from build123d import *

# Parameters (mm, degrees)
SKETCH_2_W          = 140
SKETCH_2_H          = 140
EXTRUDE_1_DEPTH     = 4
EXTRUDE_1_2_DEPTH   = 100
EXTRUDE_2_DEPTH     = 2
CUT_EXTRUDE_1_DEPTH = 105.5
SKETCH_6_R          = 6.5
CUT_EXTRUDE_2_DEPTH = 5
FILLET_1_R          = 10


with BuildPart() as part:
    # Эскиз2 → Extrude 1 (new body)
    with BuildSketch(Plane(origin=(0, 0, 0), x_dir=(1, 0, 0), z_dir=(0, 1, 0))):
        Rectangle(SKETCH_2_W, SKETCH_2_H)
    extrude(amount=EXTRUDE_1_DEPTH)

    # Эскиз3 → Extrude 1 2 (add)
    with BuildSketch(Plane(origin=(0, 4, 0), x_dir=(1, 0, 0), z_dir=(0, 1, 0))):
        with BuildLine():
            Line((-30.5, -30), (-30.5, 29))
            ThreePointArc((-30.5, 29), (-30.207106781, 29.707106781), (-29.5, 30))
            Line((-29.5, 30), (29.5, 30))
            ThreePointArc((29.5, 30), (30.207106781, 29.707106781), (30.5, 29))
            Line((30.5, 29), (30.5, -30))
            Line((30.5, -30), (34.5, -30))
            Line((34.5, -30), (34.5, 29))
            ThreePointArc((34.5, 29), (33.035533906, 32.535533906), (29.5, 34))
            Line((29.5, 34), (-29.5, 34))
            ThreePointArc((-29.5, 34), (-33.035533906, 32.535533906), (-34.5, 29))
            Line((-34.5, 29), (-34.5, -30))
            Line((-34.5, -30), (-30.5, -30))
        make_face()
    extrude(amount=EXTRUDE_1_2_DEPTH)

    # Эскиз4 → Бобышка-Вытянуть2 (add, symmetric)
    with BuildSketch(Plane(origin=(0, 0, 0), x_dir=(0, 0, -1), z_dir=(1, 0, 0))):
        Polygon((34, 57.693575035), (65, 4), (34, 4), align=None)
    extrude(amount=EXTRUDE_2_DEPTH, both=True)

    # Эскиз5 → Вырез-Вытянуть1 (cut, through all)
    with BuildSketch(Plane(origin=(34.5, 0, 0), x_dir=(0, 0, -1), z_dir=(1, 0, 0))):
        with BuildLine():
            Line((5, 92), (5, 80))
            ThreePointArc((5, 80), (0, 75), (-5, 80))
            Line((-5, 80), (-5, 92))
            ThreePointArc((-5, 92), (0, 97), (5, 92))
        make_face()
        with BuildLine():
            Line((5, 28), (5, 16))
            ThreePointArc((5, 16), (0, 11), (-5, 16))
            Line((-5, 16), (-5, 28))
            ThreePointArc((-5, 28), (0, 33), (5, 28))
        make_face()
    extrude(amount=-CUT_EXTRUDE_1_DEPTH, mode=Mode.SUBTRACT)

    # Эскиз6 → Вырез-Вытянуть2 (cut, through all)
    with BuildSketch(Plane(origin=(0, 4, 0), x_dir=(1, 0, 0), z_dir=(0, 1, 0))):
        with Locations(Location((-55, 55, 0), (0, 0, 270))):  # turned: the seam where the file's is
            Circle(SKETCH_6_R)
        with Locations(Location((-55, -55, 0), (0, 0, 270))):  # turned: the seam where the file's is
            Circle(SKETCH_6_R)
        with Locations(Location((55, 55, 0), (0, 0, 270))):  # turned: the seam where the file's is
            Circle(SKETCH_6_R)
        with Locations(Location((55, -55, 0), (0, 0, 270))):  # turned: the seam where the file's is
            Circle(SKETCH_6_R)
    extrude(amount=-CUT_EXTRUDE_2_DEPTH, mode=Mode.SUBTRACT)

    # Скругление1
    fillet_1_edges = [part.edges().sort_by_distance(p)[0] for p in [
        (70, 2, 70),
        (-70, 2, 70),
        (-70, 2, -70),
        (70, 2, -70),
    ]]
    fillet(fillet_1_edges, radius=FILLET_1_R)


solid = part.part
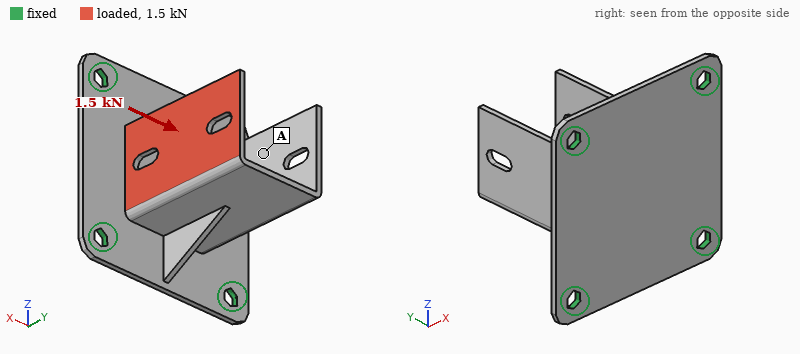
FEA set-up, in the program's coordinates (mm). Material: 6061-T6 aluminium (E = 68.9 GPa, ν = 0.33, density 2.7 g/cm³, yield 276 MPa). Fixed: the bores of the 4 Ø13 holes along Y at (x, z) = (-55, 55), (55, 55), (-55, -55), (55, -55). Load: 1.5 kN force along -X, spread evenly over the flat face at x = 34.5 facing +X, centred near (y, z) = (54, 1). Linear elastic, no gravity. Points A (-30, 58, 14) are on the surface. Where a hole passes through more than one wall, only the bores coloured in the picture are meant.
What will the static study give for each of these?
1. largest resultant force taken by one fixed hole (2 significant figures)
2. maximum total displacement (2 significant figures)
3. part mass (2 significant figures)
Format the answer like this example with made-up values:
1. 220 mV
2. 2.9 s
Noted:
1. 930 N
2. 2.0 mm
3. 410 g
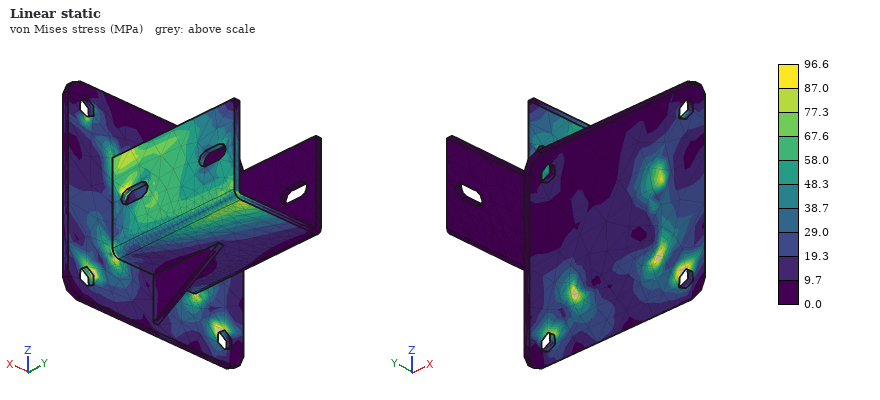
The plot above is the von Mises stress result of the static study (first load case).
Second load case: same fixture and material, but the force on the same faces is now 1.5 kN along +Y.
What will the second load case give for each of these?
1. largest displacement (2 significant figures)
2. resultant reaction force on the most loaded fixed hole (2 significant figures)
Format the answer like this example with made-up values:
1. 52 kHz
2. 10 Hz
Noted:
1. 0.23 mm
2. 690 N
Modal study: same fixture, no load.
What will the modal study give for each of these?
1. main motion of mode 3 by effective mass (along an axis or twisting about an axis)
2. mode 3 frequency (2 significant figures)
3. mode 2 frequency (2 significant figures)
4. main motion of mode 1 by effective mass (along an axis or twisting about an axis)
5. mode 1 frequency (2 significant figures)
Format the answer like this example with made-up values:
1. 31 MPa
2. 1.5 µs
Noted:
1. along Z
2. 1000 Hz
3. 860 Hz
4. along X
5. 680 Hz
